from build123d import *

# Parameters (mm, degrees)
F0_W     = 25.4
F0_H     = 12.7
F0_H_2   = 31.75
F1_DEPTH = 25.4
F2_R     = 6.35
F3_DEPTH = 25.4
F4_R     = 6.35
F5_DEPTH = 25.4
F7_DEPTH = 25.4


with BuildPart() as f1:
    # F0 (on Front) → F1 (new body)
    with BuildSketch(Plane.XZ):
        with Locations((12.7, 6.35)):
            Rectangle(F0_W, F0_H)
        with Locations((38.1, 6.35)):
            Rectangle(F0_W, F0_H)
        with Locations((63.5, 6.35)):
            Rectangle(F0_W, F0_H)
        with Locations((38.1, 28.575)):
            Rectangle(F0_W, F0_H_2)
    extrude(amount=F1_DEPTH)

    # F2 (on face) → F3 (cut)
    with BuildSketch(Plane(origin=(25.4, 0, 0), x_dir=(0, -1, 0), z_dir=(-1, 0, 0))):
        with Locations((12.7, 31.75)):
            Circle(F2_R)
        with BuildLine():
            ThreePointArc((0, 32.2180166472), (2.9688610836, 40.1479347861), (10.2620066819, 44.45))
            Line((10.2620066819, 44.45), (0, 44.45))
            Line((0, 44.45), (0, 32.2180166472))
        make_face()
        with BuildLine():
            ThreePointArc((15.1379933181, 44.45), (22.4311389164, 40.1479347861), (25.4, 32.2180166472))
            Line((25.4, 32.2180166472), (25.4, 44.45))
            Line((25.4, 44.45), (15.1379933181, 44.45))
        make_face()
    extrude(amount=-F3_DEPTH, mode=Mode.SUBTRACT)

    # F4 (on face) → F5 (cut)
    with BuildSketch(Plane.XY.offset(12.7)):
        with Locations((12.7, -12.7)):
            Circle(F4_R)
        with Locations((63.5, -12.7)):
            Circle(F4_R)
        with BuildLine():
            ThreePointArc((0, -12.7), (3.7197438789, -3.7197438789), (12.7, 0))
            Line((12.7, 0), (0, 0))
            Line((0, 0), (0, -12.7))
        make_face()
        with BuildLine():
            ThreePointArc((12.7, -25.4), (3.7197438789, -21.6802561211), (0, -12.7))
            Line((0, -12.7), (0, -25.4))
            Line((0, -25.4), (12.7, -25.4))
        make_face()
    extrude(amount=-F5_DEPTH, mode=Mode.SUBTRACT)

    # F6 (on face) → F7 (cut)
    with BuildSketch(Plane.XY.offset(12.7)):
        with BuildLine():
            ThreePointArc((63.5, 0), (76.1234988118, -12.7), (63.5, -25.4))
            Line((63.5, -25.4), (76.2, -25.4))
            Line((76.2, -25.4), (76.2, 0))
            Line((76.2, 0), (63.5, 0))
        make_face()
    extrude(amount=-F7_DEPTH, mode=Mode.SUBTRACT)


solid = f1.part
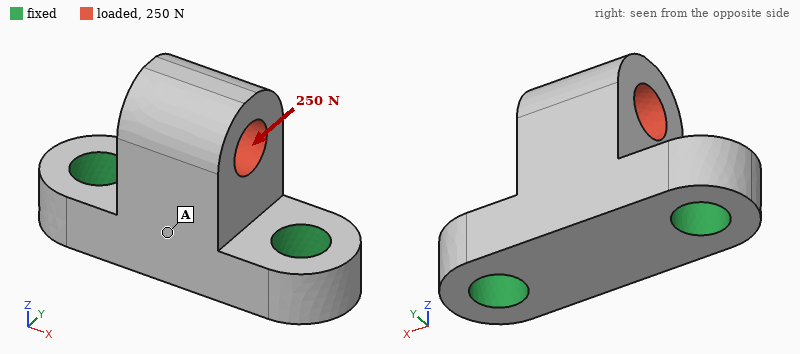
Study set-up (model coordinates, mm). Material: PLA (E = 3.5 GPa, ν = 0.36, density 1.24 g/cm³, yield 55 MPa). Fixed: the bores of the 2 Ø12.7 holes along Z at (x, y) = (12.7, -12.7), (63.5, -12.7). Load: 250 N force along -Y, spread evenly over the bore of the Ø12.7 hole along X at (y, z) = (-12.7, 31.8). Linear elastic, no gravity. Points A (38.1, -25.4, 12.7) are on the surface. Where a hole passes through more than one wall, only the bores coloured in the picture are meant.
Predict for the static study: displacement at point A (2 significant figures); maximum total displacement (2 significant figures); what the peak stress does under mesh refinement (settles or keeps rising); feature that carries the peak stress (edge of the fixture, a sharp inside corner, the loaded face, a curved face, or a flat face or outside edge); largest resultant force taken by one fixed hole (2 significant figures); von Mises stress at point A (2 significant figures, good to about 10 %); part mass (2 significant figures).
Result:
0.035 mm
0.11 mm
keeps rising
edge of the fixture
130 N
0.98 MPa
44 g
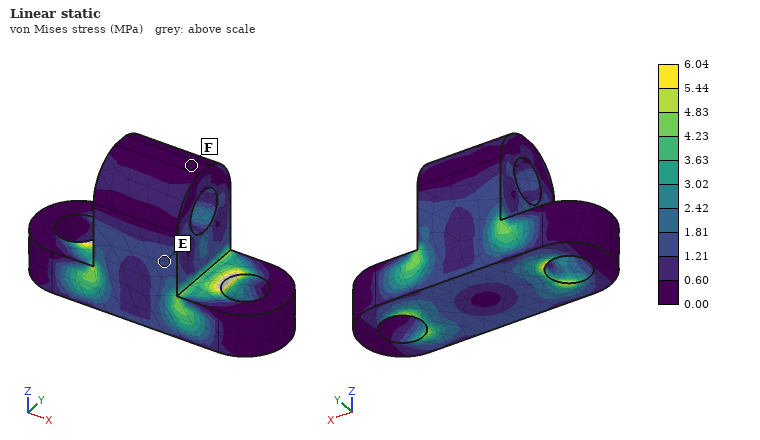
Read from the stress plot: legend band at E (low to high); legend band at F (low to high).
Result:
1.21 to 1.81 MPa
0.00 to 0.60 MPa
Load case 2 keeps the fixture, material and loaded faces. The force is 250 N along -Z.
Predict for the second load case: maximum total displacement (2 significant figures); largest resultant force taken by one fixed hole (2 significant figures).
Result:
11 µm
130 N
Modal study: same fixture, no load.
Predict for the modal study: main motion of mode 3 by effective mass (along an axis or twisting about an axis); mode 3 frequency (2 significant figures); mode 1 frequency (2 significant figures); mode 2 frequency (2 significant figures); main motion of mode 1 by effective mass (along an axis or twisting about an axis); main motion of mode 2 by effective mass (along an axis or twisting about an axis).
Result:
along Z
5600 Hz
2300 Hz
3900 Hz
along Y
along X
